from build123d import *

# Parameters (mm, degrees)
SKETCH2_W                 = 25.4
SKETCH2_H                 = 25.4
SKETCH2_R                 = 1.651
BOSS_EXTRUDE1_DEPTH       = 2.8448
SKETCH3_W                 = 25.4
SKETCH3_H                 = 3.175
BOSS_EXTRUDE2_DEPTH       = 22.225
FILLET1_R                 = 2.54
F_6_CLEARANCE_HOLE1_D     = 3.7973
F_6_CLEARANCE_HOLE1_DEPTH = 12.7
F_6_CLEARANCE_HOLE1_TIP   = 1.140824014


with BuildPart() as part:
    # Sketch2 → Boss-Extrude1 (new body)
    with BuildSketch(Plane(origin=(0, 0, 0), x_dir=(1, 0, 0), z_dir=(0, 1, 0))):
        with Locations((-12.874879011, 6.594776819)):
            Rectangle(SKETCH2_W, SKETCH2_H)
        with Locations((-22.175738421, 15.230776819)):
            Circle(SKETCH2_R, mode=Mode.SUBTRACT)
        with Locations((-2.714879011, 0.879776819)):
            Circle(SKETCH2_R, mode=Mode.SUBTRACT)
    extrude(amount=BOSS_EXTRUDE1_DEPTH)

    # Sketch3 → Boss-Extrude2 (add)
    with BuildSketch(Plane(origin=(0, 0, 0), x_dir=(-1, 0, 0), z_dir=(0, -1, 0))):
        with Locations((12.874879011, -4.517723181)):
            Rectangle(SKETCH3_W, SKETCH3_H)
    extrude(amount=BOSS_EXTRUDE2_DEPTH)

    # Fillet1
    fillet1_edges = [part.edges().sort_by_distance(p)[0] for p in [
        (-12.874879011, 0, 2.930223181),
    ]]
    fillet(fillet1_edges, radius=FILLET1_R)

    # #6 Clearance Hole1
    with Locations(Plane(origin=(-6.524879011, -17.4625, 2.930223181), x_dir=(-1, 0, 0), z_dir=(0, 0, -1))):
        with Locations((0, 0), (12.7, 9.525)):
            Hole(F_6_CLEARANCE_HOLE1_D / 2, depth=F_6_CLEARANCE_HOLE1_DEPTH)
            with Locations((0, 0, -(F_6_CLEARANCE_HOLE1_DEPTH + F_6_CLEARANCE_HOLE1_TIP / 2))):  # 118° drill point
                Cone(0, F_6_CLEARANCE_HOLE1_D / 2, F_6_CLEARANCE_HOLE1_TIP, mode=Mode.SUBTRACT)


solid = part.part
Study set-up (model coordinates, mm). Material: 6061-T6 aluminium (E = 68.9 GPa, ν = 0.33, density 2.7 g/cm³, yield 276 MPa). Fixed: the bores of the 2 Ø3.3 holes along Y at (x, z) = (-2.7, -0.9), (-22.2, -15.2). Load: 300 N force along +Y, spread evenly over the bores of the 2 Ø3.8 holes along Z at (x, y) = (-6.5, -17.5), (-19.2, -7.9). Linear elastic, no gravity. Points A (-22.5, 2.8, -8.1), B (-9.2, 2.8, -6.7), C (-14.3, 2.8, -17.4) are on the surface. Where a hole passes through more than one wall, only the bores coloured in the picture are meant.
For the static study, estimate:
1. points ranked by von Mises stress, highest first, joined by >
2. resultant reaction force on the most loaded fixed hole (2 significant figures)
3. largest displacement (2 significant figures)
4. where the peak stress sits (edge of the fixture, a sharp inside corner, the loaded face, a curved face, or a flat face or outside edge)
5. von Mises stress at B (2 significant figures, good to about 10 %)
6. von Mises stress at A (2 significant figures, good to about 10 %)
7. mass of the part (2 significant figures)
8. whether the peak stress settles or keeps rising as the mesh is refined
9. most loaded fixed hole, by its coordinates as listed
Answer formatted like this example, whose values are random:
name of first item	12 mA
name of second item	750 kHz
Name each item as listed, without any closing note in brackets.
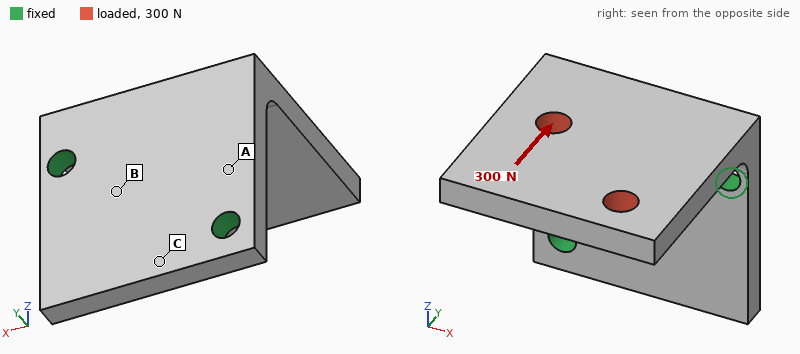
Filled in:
points ranked by von Mises stress, highest first, joined by >	A > B > C
resultant reaction force on the most loaded fixed hole	250 N
largest displacement	0.13 mm
where the peak stress sits	edge of the fixture
von Mises stress at B	20 MPa
von Mises stress at A	36 MPa
mass of the part	9.6 g
whether the peak stress settles or keeps rising as the mesh is refined	keeps rising
most loaded fixed hole, by its coordinates as listed	(-2.7, -0.9)
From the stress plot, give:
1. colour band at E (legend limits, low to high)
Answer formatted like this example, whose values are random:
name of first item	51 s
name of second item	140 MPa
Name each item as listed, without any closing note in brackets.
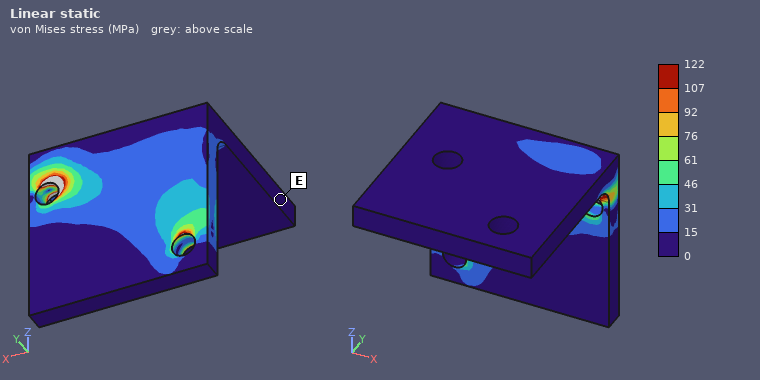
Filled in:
colour band at E	0 to 15 MPa
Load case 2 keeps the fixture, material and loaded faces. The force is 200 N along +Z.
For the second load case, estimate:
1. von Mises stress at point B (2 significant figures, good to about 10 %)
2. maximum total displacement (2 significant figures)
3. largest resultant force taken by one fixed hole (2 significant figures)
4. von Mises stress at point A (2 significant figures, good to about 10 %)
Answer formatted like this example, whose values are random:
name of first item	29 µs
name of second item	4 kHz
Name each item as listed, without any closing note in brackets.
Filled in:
von Mises stress at point B	15 MPa
maximum total displacement	0.19 mm
largest resultant force taken by one fixed hole	120 N
von Mises stress at point A	23 MPa
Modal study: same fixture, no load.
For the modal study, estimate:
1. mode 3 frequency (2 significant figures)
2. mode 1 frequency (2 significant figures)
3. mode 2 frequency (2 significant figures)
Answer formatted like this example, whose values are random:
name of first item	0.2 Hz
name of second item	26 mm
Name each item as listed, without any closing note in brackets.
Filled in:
mode 3 frequency	9500 Hz
mode 1 frequency	2900 Hz
mode 2 frequency	4800 Hz
